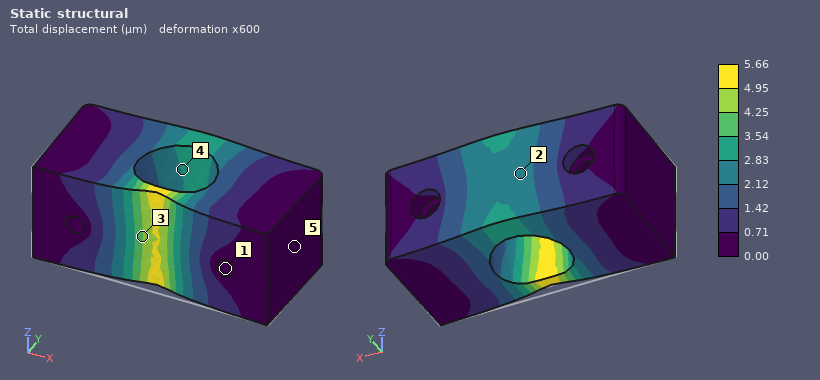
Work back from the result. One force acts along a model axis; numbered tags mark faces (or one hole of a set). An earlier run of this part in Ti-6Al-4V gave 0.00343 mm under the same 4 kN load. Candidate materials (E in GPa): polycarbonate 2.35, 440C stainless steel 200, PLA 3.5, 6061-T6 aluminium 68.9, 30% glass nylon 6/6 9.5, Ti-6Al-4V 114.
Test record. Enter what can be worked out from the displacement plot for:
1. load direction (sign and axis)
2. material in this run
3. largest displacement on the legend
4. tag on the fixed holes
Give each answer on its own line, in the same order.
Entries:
+Y
6061-T6 aluminium
5.66 µm
1
